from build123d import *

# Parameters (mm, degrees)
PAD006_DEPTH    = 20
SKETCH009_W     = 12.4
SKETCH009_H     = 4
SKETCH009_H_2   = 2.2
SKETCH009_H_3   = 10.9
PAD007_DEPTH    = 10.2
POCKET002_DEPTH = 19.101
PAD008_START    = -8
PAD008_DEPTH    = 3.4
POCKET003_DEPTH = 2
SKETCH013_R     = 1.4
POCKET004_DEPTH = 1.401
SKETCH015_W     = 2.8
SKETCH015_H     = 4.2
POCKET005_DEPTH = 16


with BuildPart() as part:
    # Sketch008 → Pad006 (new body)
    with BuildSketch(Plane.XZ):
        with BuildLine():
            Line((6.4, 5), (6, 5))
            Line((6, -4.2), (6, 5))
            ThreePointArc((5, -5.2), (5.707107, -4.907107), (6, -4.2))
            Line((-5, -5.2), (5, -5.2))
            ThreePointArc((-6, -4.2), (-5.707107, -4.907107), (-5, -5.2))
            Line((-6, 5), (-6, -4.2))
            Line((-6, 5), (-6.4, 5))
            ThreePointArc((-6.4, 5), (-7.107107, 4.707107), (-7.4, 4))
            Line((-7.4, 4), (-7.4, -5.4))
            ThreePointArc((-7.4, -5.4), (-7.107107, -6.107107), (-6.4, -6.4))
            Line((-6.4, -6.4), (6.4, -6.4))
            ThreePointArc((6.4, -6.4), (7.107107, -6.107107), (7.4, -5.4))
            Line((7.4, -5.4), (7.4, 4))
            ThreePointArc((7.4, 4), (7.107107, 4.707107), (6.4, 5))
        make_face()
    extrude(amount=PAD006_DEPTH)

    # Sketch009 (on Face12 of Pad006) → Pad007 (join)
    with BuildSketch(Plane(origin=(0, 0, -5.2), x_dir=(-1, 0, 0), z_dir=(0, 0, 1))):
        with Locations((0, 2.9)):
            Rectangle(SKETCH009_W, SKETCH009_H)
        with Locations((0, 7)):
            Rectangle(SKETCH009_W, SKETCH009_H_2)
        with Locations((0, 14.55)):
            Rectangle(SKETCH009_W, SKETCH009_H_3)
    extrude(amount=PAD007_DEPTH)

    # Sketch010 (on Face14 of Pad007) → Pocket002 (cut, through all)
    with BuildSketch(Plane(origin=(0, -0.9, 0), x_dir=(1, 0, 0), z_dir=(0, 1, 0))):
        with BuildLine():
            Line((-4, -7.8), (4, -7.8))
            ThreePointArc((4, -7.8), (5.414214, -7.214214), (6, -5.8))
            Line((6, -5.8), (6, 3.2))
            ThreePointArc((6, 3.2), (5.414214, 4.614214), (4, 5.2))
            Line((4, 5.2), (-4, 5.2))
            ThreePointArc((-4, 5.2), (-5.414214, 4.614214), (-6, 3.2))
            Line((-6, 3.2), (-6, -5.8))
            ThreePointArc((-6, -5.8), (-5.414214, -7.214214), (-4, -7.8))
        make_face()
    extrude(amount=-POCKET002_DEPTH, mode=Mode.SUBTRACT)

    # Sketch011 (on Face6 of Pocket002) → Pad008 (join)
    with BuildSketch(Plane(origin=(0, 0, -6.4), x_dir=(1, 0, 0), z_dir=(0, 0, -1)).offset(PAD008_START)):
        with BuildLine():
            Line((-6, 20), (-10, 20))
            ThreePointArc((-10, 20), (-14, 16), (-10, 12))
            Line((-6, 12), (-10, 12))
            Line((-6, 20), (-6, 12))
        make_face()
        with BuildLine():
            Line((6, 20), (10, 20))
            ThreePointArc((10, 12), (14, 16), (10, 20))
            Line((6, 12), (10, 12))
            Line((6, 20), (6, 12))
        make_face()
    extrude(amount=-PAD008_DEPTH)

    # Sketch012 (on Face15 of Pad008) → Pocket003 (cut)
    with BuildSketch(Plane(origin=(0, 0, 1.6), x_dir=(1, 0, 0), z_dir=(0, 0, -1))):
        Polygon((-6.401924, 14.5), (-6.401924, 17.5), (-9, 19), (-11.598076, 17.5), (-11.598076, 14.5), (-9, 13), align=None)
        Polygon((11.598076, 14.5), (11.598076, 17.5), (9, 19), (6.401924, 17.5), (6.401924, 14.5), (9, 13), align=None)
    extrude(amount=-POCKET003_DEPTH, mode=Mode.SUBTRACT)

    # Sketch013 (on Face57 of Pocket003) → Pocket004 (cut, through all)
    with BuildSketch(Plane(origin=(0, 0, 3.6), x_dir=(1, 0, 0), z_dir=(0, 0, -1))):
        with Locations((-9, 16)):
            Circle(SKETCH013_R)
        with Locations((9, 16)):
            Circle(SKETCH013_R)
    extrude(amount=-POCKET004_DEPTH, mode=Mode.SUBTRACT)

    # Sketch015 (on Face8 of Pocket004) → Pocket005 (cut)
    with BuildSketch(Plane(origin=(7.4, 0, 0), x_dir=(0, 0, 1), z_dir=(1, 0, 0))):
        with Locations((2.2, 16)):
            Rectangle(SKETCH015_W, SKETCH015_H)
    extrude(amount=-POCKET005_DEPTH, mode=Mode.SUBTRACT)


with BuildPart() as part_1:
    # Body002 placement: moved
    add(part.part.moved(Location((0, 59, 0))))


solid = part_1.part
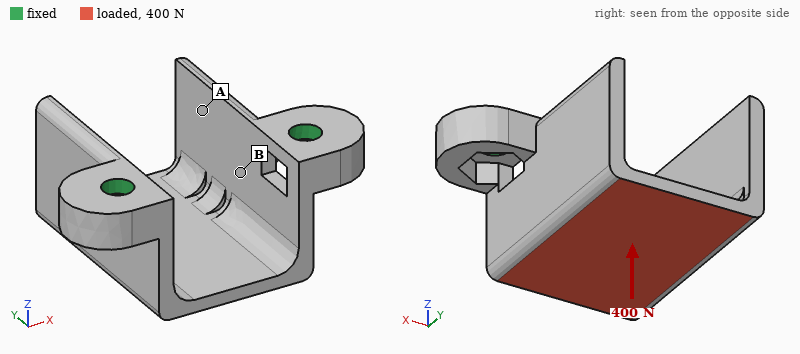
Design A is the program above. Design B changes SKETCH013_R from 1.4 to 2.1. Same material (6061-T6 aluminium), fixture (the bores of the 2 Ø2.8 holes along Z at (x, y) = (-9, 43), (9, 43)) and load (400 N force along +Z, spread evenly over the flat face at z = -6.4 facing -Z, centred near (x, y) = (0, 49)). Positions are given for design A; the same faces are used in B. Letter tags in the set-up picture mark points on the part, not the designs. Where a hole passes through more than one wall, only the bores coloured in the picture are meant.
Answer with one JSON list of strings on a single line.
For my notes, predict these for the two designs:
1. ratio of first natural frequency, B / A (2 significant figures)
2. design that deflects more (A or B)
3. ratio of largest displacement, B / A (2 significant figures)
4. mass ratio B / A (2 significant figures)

["1.2", "A", "0.69", "0.98"]
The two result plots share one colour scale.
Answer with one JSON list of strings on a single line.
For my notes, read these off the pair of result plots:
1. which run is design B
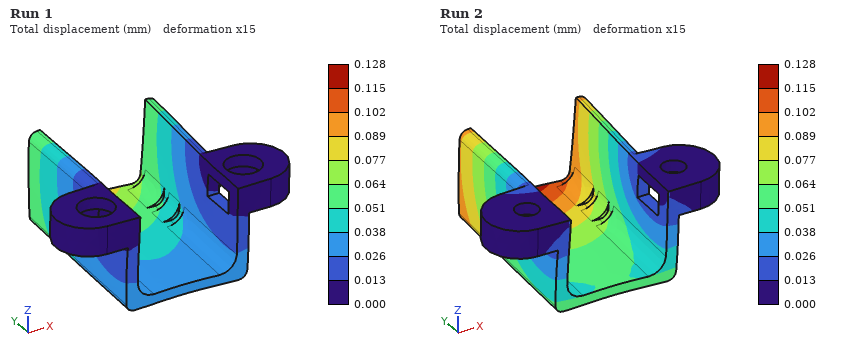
["Run 1"]
